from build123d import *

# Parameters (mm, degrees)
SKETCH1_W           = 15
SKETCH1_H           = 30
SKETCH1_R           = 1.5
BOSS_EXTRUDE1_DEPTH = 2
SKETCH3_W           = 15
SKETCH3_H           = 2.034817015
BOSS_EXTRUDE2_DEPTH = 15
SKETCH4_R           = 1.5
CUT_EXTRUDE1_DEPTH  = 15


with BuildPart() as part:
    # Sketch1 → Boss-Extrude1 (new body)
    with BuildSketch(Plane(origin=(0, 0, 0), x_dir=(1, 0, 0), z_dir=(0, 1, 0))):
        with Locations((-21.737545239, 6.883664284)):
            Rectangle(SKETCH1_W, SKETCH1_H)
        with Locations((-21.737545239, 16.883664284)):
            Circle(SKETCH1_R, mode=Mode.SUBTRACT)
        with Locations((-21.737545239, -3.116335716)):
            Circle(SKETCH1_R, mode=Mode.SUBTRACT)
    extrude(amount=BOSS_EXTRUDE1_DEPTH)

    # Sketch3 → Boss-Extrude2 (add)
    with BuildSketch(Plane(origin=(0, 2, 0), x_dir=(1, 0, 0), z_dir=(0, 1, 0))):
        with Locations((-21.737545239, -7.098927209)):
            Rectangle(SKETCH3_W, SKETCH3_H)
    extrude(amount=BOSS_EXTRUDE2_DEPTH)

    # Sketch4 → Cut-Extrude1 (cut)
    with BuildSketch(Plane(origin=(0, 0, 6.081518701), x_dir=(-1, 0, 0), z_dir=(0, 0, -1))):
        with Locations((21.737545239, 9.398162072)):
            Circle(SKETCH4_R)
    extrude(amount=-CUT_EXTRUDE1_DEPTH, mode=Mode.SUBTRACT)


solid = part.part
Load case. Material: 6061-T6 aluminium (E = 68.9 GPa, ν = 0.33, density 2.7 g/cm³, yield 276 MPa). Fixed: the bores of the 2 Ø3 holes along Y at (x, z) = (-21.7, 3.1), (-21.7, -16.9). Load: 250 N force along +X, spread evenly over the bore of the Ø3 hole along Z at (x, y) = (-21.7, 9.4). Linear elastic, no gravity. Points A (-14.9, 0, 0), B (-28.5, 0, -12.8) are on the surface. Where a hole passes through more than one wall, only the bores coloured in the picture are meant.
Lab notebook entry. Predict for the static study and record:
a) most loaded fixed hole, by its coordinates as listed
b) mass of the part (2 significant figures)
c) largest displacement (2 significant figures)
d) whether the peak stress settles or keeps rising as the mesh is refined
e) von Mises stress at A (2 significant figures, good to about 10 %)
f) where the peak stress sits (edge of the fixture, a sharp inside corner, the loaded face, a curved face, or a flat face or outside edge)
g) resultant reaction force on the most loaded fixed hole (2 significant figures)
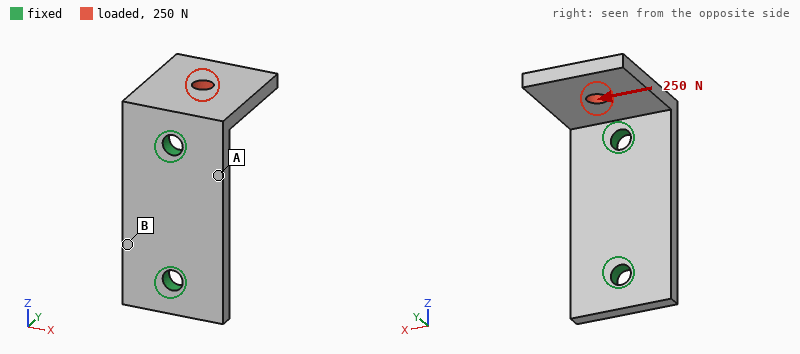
(-21.7, 3.1)
3.6 g
0.11 mm
keeps rising
45 MPa
edge of the fixture
280 N
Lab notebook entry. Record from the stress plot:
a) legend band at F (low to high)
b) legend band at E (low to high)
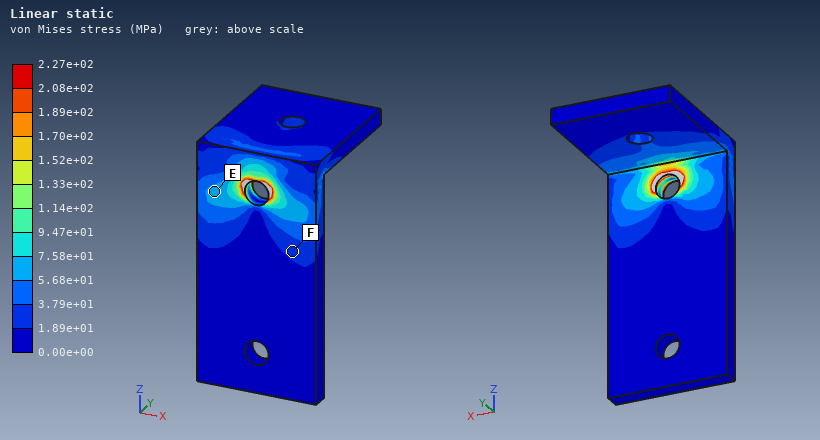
1.89e+01 to 3.79e+01 MPa
5.68e+01 to 7.58e+01 MPa
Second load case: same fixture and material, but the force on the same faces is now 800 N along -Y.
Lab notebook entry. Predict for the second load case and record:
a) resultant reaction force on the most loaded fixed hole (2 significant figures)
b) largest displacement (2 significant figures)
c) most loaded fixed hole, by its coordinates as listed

820 N
0.14 mm
(-21.7, 3.1)
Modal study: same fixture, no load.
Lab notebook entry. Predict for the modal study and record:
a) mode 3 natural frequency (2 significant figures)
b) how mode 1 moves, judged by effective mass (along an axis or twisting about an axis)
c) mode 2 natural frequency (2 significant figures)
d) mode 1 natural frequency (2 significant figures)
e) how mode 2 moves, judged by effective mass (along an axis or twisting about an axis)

14 kHz
along Z
8000 Hz
4900 Hz
along X
